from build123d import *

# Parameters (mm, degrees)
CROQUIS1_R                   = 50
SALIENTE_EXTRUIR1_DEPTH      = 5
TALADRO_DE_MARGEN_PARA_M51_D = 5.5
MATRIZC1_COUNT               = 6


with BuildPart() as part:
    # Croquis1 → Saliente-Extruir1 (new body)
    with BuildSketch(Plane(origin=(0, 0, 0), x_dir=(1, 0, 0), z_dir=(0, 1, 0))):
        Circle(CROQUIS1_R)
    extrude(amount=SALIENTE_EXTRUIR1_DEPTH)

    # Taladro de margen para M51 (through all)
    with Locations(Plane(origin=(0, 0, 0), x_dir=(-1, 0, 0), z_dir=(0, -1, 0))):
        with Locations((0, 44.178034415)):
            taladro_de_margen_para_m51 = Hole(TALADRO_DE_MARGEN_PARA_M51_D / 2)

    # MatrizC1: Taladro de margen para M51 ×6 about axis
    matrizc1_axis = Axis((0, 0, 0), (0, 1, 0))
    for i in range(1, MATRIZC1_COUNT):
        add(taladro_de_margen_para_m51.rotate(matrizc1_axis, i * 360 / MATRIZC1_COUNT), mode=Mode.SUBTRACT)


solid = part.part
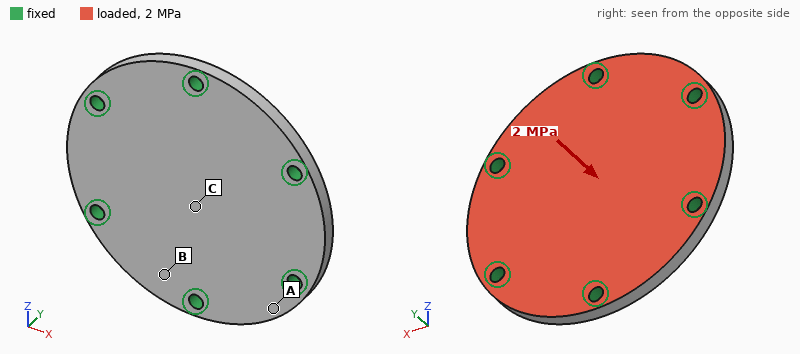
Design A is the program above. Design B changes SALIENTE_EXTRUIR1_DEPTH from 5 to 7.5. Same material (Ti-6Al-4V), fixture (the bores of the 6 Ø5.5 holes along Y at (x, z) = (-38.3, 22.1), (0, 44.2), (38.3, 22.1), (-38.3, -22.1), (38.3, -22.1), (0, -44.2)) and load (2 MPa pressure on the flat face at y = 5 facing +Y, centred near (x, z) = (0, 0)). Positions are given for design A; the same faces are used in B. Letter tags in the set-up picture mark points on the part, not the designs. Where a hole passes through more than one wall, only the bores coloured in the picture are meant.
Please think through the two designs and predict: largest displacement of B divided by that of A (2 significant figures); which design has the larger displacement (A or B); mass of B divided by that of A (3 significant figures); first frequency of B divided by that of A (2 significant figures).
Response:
0.34
A
1.50
1.4
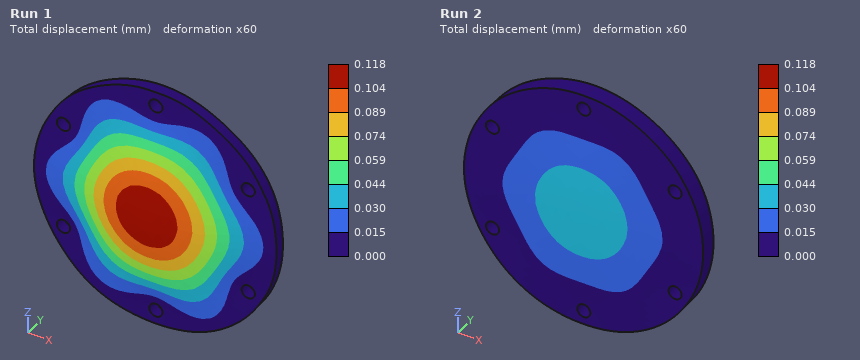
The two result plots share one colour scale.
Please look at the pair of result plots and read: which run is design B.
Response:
Run 2
